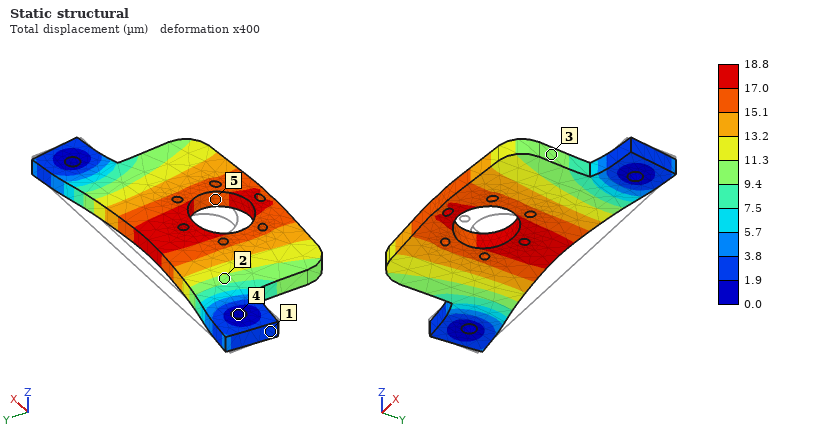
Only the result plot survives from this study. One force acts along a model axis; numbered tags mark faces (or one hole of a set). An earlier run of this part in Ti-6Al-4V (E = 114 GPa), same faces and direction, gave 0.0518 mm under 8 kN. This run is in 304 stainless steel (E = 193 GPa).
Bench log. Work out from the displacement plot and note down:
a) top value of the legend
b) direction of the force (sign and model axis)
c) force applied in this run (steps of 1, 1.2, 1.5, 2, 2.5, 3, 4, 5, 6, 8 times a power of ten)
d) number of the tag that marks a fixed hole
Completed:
18.8 µm
-Y
5 kN
4
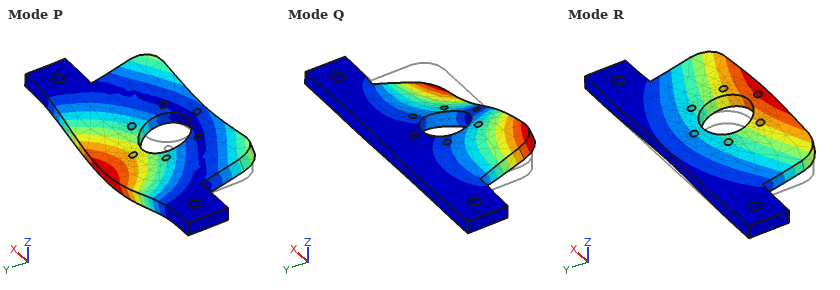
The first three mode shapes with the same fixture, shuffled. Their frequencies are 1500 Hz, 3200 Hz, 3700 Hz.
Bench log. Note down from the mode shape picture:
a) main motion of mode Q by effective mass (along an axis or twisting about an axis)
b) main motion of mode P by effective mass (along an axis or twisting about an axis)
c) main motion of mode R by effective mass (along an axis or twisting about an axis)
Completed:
twisting about Y
along Z
along Z
